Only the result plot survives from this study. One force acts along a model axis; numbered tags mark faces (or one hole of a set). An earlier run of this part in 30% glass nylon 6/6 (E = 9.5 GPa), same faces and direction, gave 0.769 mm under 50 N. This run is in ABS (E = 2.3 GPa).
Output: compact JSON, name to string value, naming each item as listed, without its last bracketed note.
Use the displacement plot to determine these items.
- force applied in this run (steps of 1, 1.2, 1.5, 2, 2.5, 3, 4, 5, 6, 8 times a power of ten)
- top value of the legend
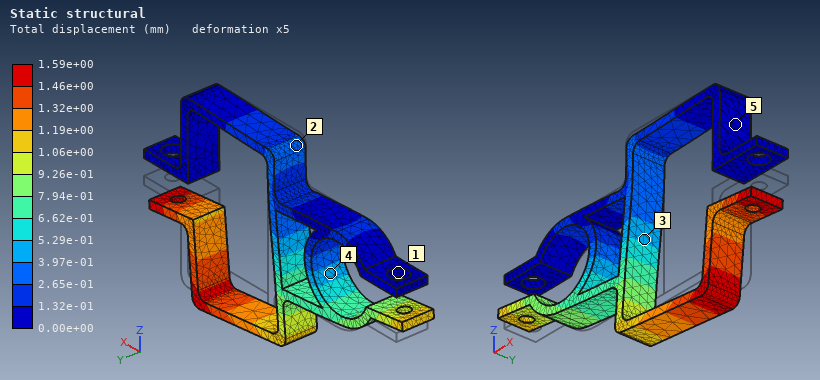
{"force applied in this run": "25 N", "top value of the legend": "1.59e+00 mm"}
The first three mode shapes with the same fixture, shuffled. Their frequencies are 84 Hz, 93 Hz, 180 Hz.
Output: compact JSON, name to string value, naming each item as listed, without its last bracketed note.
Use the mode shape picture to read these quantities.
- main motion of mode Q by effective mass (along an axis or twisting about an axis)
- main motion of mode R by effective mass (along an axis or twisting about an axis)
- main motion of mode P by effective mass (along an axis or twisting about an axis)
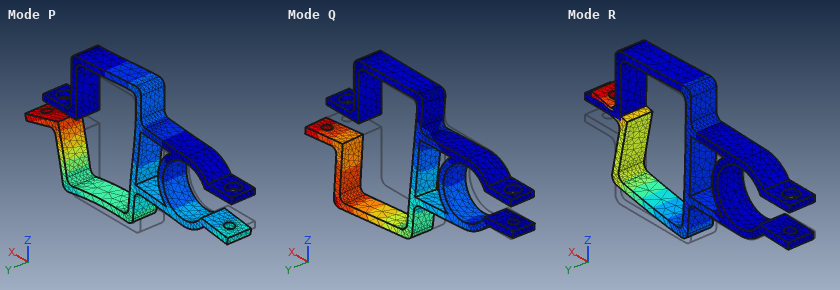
{"main motion of mode Q by effective mass": "along Y", "main motion of mode R by effective mass": "along Z", "main motion of mode P by effective mass": "along X"}
